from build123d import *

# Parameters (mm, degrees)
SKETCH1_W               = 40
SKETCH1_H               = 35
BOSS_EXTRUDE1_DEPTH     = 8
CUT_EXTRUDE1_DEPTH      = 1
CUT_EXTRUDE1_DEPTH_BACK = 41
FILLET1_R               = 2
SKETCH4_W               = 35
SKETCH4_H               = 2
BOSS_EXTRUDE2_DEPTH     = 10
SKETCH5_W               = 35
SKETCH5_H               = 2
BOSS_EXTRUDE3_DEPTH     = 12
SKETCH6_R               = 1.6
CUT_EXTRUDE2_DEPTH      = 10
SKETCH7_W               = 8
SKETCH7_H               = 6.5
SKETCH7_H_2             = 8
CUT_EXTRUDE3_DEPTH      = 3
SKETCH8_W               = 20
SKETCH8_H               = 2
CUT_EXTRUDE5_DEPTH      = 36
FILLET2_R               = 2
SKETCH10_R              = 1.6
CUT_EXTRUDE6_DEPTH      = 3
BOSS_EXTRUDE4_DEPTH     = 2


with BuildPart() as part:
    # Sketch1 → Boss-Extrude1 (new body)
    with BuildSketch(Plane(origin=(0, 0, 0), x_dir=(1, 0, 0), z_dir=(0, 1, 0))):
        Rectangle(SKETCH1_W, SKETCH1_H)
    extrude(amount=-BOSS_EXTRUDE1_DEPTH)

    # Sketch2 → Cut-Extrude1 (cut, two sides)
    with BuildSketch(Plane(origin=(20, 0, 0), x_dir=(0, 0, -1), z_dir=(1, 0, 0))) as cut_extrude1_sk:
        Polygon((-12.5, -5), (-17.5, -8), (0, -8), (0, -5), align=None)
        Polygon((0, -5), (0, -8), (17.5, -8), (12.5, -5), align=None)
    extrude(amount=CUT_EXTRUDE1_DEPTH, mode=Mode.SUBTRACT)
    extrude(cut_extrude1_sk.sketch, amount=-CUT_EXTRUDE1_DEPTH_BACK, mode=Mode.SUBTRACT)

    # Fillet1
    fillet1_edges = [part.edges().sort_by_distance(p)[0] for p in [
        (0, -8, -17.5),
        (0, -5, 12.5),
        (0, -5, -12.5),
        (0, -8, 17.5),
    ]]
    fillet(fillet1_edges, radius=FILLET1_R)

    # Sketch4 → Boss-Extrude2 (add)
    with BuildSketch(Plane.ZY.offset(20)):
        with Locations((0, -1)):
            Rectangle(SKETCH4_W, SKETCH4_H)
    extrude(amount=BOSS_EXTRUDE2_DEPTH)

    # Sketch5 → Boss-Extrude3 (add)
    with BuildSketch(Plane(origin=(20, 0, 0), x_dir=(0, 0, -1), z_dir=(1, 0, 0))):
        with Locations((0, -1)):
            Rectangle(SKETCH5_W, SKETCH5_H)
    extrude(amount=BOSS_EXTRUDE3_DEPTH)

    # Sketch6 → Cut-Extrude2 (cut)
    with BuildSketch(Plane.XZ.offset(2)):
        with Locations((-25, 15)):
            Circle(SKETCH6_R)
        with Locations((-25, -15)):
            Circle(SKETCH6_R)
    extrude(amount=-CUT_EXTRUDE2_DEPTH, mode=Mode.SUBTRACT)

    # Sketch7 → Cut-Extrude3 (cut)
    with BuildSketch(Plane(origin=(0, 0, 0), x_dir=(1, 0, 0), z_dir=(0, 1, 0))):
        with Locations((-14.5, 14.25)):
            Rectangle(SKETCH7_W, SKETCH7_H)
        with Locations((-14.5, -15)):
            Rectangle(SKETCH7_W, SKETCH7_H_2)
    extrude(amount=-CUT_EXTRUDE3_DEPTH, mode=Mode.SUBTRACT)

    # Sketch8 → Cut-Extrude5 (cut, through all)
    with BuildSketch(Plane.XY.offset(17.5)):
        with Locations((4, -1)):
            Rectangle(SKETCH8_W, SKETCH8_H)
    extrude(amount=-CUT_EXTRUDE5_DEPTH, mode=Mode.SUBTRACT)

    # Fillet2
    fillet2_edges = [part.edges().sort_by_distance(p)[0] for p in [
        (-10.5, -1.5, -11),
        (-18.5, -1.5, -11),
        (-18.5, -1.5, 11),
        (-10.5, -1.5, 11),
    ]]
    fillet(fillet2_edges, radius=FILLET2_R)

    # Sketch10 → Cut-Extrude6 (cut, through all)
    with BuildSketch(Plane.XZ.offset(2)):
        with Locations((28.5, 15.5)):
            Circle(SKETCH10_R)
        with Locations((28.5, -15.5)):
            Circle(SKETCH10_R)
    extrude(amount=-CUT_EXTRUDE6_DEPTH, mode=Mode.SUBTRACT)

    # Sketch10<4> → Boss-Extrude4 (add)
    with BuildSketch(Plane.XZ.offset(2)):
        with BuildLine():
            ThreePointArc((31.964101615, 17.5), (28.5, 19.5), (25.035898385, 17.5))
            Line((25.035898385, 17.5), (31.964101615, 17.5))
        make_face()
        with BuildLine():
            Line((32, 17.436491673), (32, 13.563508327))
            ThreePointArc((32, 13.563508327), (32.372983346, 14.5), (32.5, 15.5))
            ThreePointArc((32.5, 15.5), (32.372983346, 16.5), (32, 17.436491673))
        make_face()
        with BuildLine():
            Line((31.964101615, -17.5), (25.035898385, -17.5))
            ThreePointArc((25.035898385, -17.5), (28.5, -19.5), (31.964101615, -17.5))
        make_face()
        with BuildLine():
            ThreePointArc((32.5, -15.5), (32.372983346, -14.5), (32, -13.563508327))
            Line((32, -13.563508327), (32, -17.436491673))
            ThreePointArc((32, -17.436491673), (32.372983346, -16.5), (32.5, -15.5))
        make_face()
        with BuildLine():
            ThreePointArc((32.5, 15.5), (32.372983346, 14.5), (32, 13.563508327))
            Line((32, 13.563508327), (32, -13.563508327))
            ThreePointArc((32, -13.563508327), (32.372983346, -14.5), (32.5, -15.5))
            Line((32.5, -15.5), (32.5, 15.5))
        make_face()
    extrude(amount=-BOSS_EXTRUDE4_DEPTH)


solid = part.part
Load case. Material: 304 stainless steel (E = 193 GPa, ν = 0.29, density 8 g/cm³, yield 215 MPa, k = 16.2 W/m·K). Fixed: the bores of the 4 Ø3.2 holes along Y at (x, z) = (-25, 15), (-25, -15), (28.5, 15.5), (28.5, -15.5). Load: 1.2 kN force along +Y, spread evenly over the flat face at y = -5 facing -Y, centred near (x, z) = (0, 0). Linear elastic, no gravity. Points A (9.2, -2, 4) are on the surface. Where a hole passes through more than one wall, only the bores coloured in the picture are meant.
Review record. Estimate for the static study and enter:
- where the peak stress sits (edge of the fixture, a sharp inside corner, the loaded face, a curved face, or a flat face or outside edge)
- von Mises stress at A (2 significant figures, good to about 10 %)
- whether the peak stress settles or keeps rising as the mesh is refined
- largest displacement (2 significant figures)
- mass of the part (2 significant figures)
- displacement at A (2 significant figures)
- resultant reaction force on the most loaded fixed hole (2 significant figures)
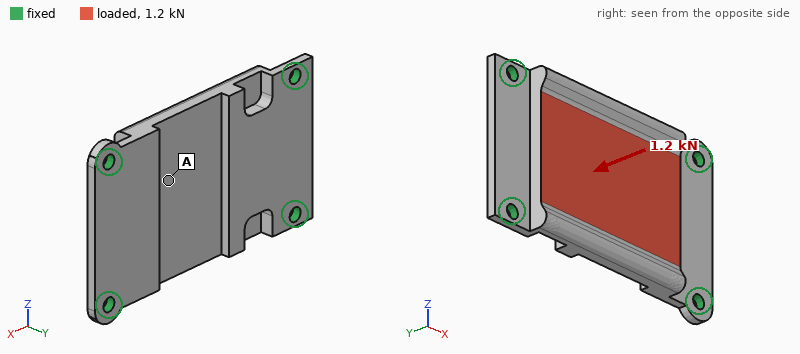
edge of the fixture
24 MPa
keeps rising
36 µm
58 g
33 µm
860 N
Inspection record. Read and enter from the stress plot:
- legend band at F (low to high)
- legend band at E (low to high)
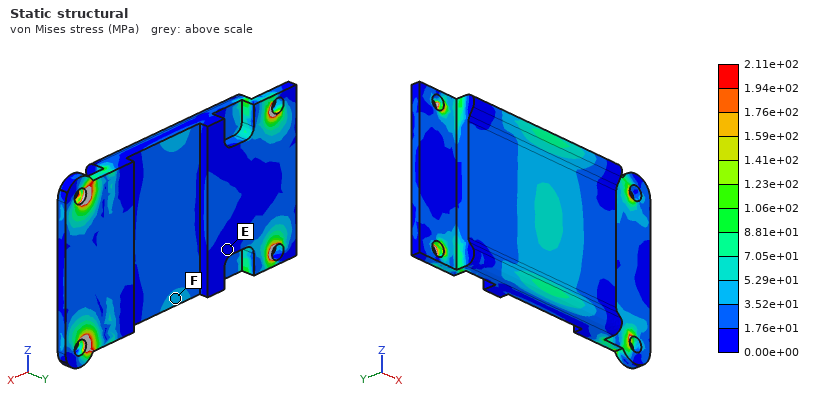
3.52e+01 to 5.29e+01 MPa
0.00e+00 to 1.76e+01 MPa
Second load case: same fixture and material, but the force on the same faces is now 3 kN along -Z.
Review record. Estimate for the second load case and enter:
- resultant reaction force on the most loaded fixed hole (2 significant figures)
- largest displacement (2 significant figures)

1.1 kN
18 µm
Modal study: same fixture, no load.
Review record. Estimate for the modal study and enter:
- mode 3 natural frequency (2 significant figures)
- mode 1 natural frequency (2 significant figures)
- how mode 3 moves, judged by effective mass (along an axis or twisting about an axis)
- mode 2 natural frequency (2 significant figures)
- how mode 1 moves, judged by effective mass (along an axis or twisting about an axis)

10 kHz
5000 Hz
twisting about Z
8000 Hz
along Y
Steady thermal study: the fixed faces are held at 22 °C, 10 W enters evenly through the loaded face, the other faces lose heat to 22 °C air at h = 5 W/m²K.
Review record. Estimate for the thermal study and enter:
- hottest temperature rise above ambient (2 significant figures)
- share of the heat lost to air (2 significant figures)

73 K
10 %
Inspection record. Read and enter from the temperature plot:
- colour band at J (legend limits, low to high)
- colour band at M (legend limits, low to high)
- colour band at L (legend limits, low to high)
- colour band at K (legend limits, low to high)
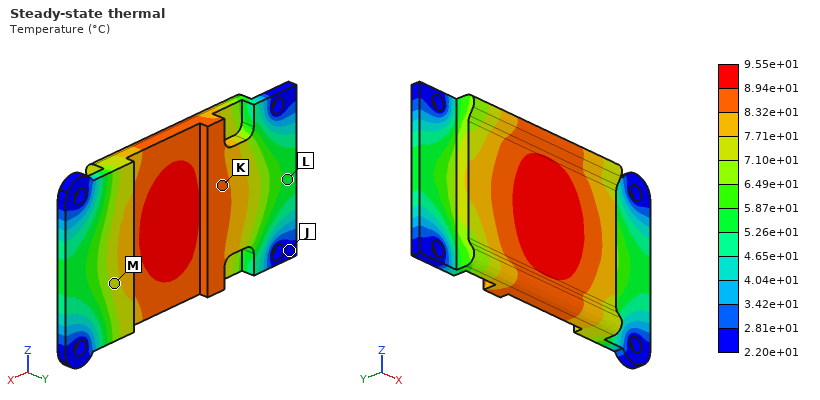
2.20e+01 to 2.81e+01 °C
7.10e+01 to 7.71e+01 °C
5.26e+01 to 5.87e+01 °C
8.32e+01 to 8.94e+01 °C
